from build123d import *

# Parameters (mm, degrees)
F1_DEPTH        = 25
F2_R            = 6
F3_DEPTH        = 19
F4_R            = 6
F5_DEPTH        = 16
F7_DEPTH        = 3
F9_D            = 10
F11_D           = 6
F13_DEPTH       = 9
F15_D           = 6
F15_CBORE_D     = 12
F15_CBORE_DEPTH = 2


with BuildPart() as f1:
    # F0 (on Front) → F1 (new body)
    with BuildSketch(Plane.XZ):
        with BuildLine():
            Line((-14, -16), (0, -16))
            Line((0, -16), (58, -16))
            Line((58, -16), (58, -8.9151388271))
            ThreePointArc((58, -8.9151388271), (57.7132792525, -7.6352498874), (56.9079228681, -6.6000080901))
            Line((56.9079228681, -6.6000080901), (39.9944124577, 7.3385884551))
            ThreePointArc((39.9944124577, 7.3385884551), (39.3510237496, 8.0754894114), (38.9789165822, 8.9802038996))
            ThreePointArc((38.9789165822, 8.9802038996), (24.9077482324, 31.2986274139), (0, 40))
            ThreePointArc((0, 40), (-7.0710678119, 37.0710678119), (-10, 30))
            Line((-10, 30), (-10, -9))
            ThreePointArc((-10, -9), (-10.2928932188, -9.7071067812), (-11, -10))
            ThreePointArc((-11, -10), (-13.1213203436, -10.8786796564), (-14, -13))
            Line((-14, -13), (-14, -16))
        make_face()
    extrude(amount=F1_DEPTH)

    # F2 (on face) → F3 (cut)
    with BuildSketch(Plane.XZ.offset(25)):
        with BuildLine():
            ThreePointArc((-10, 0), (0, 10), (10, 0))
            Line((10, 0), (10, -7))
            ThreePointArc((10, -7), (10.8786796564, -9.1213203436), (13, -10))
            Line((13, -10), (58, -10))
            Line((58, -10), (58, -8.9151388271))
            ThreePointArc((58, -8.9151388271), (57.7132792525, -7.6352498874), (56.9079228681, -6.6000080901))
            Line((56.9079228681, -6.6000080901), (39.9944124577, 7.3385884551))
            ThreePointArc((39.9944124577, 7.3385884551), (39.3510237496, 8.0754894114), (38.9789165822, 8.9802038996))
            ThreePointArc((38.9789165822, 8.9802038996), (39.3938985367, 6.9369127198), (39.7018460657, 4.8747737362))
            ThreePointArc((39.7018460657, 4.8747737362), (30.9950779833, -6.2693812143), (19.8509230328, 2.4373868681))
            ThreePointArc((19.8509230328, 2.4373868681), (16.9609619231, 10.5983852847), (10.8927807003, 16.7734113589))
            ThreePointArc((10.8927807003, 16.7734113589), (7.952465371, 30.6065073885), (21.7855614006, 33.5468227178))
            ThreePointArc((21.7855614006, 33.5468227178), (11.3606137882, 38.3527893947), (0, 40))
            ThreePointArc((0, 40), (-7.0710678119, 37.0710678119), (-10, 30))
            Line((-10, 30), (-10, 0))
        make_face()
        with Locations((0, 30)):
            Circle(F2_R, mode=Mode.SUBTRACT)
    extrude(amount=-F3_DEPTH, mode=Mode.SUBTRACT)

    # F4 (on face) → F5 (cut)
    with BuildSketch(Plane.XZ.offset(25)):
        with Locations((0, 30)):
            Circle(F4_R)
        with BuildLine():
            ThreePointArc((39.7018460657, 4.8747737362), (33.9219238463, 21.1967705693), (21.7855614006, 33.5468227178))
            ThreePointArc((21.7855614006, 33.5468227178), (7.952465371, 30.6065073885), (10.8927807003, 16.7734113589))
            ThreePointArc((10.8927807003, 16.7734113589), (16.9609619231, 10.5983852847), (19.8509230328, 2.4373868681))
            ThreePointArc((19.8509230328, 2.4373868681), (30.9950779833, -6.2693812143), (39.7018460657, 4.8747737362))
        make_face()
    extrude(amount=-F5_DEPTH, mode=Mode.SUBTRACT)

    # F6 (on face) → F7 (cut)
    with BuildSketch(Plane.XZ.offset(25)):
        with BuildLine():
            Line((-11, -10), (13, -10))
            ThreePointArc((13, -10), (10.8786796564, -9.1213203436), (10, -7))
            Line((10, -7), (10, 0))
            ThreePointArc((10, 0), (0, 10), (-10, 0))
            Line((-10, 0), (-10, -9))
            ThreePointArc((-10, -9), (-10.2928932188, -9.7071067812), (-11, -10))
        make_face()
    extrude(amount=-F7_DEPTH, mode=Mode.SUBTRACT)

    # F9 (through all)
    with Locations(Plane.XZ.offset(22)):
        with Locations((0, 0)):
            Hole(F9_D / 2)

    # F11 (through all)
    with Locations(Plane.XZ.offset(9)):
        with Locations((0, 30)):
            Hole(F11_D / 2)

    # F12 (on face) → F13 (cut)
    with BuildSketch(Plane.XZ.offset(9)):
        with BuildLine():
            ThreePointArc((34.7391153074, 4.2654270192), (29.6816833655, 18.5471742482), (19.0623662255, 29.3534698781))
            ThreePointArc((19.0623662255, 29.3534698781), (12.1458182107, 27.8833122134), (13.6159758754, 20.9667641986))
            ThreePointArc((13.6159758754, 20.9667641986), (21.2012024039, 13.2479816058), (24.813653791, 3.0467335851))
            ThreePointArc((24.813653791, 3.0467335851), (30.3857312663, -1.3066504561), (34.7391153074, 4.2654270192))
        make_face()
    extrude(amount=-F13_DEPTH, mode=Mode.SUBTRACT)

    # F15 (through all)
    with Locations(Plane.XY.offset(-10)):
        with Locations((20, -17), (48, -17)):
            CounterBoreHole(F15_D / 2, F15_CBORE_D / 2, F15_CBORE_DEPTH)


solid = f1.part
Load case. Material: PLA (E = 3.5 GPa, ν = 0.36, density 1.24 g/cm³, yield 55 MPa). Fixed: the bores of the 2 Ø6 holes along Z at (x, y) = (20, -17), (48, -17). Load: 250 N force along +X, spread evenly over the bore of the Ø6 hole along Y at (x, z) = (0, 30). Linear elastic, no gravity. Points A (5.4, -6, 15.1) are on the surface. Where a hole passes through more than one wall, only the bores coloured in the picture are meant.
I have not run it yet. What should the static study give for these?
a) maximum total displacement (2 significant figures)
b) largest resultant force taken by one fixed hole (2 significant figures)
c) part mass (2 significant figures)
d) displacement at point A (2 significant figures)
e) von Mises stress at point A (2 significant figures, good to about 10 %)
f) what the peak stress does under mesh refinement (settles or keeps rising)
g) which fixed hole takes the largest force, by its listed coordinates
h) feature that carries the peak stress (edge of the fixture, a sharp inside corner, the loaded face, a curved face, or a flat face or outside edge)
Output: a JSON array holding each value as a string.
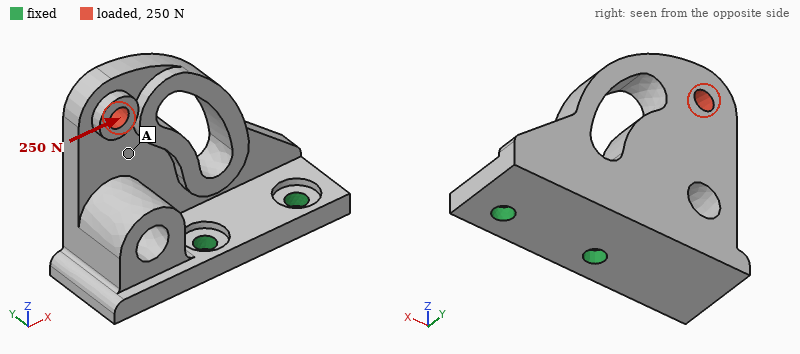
["1.1 mm", "390 N", "34 g", "0.62 mm", "5.6 MPa", "keeps rising", "(48, -17)", "edge of the fixture"]
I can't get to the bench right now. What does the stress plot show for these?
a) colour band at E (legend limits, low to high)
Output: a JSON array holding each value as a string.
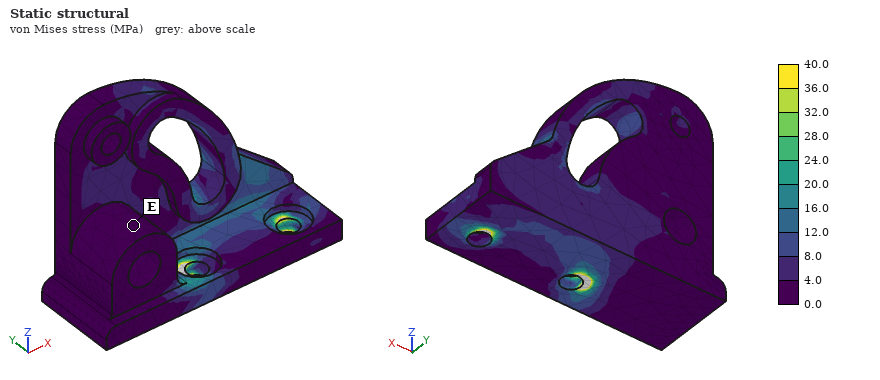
["0.0 to 4.0 MPa"]
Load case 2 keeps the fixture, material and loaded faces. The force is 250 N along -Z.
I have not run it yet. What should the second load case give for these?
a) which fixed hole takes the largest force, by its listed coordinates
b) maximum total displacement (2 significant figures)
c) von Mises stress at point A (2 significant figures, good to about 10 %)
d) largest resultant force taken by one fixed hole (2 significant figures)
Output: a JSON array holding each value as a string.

["(20, -17)", "1.1 mm", "4.6 MPa", "380 N"]
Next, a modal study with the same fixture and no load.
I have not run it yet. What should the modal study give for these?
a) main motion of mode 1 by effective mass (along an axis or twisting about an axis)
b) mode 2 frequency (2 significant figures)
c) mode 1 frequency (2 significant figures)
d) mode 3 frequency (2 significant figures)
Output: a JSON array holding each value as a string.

["along Y", "950 Hz", "520 Hz", "2000 Hz"]
